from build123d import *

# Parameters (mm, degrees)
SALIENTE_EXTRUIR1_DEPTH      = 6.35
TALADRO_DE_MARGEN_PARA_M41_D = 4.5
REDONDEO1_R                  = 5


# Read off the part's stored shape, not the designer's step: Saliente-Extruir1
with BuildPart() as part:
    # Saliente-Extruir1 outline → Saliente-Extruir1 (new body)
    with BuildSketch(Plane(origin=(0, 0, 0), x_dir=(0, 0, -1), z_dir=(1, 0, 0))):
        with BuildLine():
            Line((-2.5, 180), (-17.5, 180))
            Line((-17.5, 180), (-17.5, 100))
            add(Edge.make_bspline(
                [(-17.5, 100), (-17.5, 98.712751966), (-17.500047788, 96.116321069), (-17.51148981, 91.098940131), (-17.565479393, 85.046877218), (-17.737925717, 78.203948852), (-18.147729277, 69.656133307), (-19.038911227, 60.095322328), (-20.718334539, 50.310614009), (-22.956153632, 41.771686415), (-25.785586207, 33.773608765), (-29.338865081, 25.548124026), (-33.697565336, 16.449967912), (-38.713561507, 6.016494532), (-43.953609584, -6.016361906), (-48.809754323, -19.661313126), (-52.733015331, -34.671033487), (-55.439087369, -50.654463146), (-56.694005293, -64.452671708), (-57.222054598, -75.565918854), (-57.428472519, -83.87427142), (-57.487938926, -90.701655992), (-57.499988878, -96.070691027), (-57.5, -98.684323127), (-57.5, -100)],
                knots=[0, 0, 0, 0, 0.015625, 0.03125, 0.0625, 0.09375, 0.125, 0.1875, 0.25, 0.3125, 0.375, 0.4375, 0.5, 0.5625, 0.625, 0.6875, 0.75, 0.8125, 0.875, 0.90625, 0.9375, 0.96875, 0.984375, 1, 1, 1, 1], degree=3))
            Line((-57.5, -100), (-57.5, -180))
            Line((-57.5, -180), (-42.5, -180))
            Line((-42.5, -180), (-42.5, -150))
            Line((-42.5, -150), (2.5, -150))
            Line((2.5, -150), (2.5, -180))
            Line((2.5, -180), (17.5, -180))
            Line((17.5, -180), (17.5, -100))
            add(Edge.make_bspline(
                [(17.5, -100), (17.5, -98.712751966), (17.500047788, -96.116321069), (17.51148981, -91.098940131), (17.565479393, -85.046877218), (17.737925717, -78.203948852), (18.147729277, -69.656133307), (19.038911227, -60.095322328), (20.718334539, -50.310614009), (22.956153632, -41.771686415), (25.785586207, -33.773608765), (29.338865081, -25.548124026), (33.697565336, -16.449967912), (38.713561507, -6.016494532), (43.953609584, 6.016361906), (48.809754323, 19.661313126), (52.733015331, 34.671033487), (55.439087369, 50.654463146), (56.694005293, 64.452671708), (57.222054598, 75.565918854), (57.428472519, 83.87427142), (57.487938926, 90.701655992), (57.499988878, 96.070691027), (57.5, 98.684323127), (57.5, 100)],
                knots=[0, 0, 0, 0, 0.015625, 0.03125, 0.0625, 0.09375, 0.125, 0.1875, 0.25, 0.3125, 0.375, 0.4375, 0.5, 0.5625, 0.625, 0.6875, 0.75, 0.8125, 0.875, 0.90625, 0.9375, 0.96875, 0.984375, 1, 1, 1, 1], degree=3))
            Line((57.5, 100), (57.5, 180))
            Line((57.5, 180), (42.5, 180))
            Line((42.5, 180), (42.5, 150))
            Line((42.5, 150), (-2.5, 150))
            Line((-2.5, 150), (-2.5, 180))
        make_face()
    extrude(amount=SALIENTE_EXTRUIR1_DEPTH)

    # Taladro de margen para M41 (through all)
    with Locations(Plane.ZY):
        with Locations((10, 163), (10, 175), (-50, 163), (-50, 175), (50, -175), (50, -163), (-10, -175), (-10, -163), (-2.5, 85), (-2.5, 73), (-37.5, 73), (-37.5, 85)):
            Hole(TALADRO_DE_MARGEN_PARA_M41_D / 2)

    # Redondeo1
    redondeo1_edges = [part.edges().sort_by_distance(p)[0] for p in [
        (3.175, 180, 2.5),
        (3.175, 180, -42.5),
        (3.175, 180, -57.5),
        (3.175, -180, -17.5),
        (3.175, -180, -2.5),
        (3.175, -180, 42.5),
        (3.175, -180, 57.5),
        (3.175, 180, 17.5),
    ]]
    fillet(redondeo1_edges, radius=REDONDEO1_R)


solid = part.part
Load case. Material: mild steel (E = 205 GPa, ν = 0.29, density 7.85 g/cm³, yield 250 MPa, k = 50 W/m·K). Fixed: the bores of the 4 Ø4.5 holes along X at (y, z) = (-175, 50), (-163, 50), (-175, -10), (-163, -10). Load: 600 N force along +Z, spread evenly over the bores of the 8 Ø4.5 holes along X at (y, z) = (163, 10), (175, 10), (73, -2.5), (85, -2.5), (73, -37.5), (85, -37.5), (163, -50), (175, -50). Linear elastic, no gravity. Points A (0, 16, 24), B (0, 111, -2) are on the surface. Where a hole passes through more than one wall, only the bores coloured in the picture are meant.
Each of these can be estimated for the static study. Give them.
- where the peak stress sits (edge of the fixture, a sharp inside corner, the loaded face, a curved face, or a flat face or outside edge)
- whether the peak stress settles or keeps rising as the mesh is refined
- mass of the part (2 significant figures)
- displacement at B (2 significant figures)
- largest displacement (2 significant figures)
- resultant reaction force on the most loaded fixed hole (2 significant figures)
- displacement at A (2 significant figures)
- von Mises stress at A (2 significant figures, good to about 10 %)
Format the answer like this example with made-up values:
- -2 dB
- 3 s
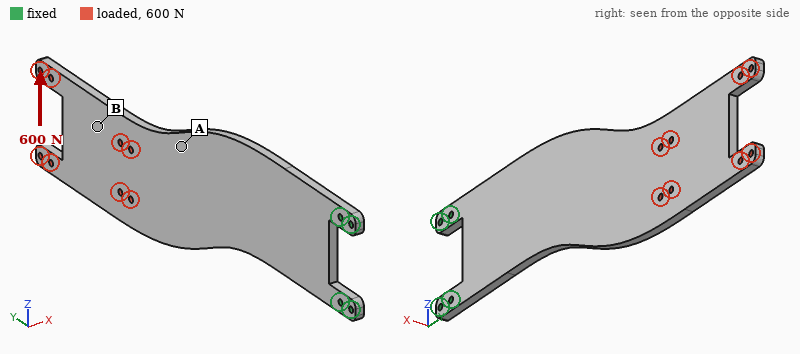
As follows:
- edge of the fixture
- keeps rising
- 1.2 kg
- 0.11 mm
- 0.16 mm
- 2.4 kN
- 0.056 mm
- 9.8 MPa
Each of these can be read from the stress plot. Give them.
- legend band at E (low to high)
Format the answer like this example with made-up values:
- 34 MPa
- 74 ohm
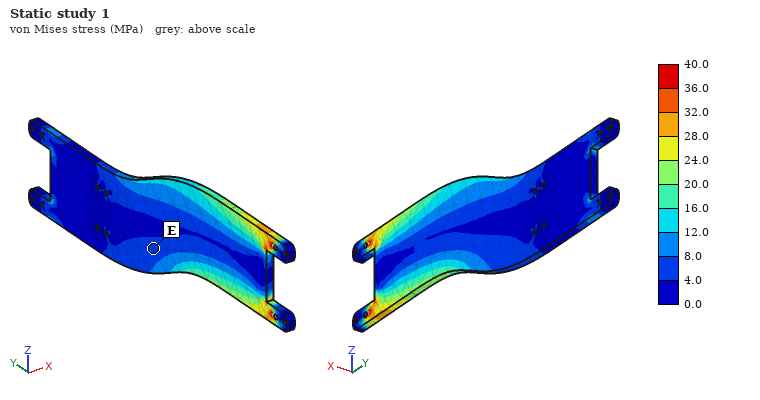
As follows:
- 4.0 to 8.0 MPa
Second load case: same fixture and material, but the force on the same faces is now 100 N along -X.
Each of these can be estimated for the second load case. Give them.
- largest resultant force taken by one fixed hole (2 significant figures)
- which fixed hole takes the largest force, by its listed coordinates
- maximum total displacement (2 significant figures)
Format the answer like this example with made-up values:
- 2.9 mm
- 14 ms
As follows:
- 370 N
- (-163, -10)
- 4.1 mm
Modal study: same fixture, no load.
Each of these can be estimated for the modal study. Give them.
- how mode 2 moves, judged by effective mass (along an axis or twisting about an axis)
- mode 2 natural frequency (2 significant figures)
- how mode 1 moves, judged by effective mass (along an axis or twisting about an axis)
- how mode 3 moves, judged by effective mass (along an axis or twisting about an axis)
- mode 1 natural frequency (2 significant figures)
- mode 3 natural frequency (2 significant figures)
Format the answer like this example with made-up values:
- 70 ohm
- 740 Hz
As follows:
- along X
- 270 Hz
- along X
- twisting about Y
- 42 Hz
- 380 Hz
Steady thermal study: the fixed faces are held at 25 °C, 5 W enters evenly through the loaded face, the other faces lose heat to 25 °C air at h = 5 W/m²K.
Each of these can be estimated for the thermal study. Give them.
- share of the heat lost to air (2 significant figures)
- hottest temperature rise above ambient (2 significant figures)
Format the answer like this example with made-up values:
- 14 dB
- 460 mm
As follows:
- 75 %
- 32 K
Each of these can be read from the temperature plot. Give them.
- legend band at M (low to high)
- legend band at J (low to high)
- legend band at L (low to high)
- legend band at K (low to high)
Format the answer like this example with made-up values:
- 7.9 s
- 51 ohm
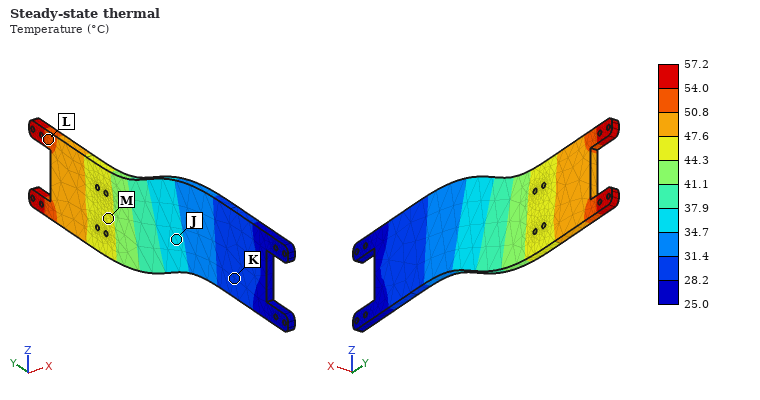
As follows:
- 44.3 to 47.6 °C
- 34.7 to 37.9 °C
- 50.8 to 54.0 °C
- 28.2 to 31.4 °C
